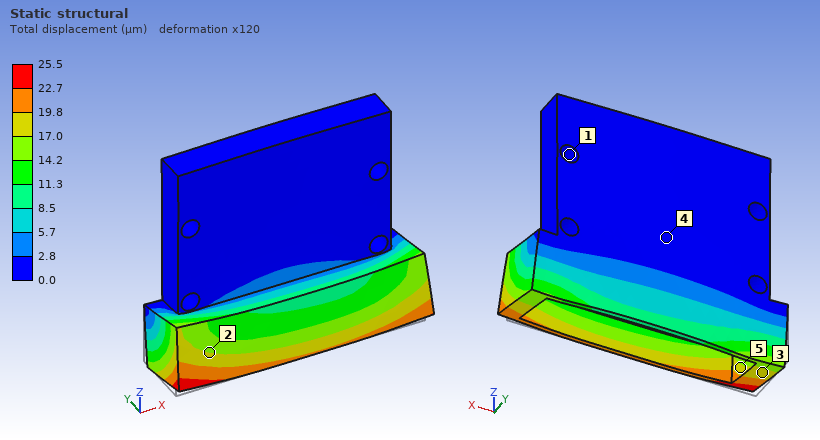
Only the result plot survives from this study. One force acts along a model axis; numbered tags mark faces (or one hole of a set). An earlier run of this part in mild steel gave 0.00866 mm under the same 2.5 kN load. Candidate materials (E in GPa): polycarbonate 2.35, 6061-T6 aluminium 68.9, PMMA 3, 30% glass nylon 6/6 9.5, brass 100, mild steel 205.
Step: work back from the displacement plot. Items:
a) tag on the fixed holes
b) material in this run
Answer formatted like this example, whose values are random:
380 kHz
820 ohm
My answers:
1
6061-T6 aluminium
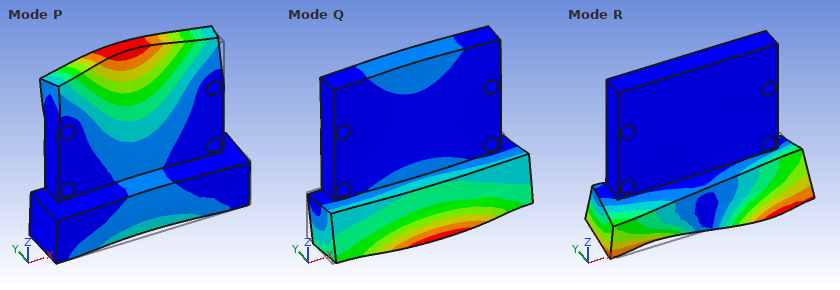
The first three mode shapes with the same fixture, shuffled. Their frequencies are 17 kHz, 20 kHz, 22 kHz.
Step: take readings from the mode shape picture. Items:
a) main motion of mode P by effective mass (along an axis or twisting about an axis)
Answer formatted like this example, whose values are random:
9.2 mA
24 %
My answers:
along Y
